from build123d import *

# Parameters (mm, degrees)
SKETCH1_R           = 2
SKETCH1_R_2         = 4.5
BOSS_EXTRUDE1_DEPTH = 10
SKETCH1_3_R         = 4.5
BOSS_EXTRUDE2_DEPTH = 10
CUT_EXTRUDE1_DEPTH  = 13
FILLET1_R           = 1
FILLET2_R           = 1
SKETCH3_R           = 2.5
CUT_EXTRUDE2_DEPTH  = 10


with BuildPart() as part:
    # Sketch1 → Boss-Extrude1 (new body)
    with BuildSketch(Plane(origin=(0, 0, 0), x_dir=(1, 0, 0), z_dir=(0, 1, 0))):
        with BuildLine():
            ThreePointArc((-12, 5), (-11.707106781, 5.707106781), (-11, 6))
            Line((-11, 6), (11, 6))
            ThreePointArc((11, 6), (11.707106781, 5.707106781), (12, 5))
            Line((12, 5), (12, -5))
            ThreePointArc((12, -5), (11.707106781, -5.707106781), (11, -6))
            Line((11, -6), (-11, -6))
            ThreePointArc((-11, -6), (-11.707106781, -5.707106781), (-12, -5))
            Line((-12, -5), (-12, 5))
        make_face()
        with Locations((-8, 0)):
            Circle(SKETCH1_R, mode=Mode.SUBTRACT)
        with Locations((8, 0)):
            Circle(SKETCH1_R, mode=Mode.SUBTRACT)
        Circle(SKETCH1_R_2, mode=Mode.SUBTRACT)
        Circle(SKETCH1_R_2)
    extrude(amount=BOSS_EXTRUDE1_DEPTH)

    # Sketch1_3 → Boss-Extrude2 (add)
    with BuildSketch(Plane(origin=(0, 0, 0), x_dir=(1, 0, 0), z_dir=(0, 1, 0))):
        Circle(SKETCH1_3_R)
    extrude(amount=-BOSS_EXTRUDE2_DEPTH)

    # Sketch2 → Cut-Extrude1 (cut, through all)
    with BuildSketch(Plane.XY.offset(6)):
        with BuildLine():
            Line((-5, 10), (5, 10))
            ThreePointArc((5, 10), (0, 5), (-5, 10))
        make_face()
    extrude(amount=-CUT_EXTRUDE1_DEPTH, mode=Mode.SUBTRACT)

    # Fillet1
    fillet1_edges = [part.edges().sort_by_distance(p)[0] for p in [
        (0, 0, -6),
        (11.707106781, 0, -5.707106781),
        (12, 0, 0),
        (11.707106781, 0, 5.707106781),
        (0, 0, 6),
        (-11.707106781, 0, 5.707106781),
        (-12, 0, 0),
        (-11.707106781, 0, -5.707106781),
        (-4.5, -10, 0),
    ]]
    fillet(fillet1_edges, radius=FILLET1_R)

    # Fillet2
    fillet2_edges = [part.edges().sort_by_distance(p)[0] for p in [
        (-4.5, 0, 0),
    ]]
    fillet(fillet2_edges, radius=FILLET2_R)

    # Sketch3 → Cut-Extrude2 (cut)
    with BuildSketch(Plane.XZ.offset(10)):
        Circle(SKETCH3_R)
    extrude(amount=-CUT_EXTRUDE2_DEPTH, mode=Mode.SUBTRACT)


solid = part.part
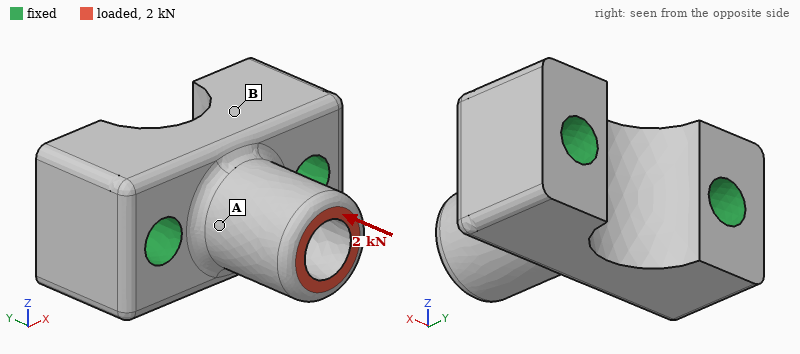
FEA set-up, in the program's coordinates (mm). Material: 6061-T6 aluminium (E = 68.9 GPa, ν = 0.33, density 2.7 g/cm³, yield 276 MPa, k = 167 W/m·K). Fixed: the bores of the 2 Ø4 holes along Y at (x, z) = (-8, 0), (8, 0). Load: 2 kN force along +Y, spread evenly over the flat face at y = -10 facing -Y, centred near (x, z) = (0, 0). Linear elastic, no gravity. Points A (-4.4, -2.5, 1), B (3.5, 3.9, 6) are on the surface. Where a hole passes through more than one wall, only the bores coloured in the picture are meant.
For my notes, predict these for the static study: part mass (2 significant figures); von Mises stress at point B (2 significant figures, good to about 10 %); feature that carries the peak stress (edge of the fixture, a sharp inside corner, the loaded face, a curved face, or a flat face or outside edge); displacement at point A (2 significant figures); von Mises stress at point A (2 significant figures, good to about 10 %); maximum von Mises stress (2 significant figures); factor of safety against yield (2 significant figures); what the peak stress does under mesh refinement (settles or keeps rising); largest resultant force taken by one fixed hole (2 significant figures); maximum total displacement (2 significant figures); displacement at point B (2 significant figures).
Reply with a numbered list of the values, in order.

1. 7.0 g
2. 18 MPa
3. a curved face
4. 4.6 µm
5. 52 MPa
6. 120 MPa
7. 2.4
8. settles
9. 1.1 kN
10. 12 µm
11. 1.9 µm
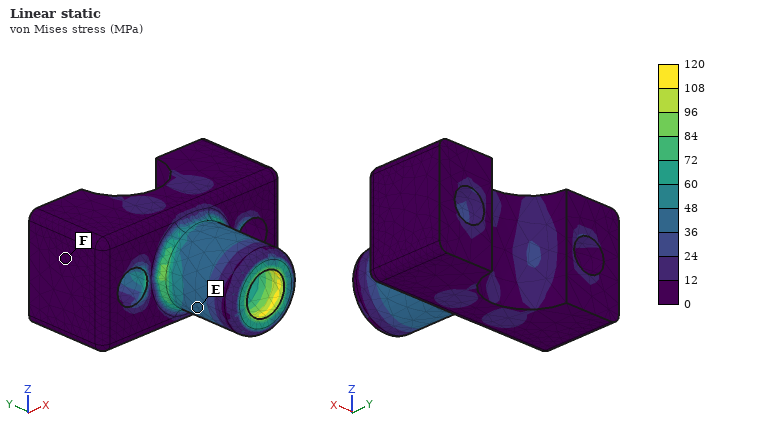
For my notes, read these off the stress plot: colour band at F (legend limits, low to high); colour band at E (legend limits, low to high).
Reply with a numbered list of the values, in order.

1. 0 to 12 MPa
2. 36 to 48 MPa
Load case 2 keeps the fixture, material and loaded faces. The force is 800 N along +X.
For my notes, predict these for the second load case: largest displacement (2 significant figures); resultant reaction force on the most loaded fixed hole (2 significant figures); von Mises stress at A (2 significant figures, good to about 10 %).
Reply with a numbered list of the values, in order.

1. 35 µm
2. 930 N
3. 94 MPa
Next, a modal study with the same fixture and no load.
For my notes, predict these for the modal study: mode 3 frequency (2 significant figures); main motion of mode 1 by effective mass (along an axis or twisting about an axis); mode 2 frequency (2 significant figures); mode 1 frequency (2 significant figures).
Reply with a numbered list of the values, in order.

1. 71 kHz
2. along Z
3. 41 kHz
4. 33 kHz
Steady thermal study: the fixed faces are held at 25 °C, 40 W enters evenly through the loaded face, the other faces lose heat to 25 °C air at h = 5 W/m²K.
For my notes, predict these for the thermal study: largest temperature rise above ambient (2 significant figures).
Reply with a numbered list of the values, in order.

1. 71 K
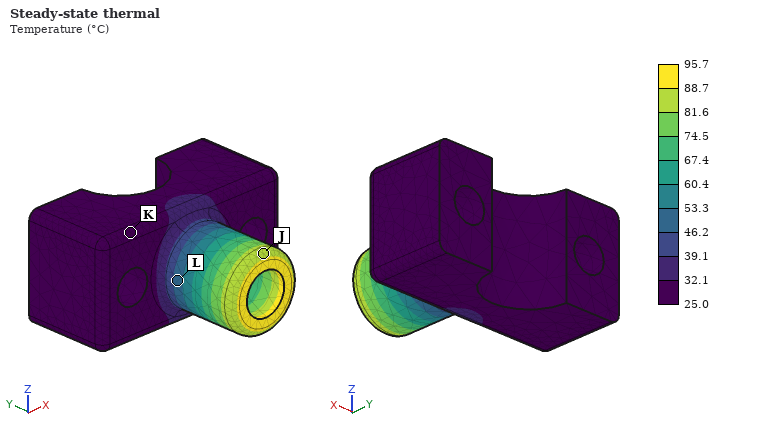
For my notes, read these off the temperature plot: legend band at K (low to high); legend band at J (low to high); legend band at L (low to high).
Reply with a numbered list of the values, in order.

1. 25.0 to 32.1 °C
2. 81.6 to 88.7 °C
3. 46.2 to 53.3 °C
